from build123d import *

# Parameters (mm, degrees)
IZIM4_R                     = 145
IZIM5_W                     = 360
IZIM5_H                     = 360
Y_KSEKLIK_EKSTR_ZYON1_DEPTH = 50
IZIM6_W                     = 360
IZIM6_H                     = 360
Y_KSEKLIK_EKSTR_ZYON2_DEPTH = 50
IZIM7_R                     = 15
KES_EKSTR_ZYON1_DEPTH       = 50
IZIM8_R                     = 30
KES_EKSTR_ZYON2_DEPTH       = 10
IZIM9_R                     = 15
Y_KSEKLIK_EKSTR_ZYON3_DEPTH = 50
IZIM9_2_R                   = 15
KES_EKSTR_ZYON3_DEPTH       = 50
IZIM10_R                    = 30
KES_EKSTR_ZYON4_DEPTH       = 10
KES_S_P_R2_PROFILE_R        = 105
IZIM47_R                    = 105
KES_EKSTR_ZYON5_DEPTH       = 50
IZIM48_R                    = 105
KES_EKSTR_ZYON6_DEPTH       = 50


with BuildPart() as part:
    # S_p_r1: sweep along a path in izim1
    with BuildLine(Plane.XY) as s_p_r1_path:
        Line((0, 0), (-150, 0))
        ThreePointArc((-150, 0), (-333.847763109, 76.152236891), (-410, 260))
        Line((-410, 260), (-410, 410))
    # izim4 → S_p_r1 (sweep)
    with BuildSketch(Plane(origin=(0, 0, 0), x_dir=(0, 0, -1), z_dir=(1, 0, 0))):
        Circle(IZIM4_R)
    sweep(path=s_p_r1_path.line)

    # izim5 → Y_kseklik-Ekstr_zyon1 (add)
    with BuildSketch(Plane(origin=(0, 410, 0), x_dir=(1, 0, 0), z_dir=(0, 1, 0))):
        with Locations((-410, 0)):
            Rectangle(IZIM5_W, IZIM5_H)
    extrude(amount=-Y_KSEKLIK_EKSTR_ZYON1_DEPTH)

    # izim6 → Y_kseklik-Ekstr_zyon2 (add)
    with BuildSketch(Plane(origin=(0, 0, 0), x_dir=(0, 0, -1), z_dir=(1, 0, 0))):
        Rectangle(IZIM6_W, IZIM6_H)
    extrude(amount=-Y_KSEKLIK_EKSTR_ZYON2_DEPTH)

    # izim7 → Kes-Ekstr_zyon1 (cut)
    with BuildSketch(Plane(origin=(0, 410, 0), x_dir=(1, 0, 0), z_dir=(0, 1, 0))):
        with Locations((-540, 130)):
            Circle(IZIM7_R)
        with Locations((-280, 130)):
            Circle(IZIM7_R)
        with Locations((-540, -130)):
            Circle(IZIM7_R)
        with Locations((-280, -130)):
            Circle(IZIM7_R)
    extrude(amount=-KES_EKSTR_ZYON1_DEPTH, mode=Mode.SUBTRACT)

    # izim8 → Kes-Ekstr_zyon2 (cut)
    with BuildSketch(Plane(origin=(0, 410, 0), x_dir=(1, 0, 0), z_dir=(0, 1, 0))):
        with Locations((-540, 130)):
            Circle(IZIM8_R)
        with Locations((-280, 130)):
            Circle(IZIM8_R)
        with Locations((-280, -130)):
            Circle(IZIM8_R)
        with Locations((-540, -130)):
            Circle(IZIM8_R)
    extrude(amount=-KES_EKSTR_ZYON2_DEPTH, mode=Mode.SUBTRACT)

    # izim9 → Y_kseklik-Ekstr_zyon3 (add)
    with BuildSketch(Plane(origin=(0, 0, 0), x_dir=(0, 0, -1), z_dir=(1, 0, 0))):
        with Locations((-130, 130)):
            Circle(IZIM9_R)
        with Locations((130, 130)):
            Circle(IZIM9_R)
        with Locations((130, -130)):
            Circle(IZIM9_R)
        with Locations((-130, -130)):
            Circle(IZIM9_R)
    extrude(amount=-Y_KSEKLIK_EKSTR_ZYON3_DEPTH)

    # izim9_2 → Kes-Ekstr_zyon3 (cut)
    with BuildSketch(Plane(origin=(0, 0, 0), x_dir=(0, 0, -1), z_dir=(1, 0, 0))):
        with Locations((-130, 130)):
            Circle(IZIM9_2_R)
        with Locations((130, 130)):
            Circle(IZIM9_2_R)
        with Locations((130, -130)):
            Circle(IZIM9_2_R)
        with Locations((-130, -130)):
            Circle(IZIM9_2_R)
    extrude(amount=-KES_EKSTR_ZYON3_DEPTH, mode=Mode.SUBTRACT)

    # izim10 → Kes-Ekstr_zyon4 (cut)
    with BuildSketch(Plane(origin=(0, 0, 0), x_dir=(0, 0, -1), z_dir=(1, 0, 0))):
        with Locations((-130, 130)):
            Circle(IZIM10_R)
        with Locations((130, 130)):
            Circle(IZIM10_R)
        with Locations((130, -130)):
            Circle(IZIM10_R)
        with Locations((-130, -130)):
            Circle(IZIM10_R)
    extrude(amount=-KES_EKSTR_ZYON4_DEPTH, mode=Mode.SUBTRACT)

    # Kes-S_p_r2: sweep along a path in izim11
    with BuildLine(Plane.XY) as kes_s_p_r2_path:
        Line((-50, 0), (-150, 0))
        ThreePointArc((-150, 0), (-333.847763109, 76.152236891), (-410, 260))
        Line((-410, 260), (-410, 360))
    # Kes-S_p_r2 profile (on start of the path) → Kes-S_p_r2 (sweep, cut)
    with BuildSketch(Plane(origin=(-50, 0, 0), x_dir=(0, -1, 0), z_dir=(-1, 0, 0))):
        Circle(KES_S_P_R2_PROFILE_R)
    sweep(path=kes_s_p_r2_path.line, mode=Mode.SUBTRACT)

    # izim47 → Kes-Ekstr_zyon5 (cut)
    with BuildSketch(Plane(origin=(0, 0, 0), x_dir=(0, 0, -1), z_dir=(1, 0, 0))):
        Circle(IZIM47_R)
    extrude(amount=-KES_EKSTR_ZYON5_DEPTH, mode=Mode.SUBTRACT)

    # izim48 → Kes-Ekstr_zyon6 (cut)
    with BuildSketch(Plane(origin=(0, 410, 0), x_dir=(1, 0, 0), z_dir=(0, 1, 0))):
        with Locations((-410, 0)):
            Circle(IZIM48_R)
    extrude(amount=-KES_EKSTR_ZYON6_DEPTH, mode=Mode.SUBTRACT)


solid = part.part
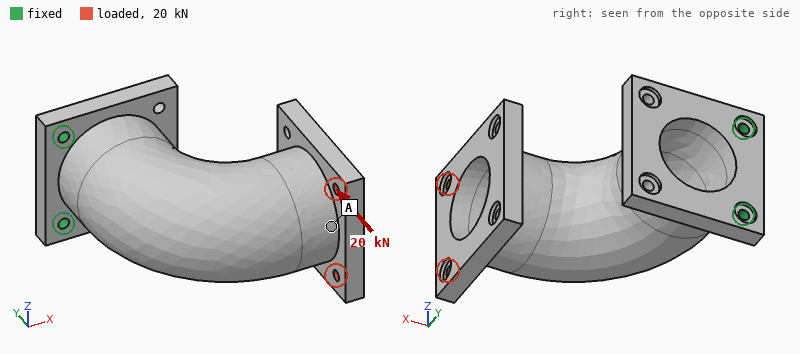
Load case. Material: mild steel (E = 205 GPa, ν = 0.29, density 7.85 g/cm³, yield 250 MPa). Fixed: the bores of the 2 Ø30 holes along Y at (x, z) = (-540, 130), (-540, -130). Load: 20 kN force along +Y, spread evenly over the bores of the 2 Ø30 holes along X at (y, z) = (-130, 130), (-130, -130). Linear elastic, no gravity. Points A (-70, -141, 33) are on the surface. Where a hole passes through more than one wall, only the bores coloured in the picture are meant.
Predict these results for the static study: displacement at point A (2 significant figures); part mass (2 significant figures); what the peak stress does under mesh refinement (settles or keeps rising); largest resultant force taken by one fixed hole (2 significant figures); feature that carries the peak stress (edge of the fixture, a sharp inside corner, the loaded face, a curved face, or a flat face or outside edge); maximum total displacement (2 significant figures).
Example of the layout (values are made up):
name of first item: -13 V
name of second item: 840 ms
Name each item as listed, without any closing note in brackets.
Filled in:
displacement at point A: 0.93 mm
part mass: 220 kg
what the peak stress does under mesh refinement: keeps rising
largest resultant force taken by one fixed hole: 10 kN
feature that carries the peak stress: edge of the fixture
maximum total displacement: 1.0 mm
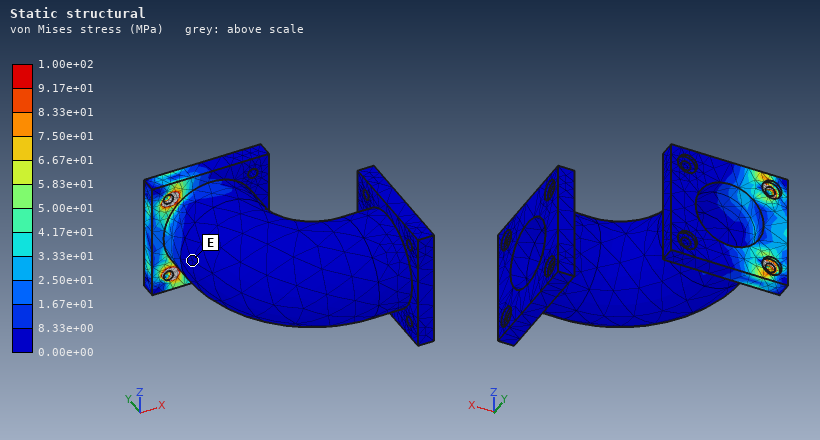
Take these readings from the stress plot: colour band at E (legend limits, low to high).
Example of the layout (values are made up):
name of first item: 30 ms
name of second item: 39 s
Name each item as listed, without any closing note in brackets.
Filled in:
colour band at E: 0.00e+00 to 8.33e+00 MPa
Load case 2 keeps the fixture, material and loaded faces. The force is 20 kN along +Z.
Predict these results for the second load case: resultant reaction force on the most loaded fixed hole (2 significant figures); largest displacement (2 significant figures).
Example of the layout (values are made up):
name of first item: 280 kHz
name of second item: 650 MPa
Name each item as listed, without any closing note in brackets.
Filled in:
resultant reaction force on the most loaded fixed hole: 56 kN
largest displacement: 0.17 mm
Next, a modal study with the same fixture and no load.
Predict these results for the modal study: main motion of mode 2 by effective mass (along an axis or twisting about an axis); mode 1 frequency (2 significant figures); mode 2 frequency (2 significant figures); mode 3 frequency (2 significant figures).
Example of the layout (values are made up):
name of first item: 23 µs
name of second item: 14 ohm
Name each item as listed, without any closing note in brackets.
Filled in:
main motion of mode 2 by effective mass: along Z
mode 1 frequency: 69 Hz
mode 2 frequency: 220 Hz
mode 3 frequency: 550 Hz
